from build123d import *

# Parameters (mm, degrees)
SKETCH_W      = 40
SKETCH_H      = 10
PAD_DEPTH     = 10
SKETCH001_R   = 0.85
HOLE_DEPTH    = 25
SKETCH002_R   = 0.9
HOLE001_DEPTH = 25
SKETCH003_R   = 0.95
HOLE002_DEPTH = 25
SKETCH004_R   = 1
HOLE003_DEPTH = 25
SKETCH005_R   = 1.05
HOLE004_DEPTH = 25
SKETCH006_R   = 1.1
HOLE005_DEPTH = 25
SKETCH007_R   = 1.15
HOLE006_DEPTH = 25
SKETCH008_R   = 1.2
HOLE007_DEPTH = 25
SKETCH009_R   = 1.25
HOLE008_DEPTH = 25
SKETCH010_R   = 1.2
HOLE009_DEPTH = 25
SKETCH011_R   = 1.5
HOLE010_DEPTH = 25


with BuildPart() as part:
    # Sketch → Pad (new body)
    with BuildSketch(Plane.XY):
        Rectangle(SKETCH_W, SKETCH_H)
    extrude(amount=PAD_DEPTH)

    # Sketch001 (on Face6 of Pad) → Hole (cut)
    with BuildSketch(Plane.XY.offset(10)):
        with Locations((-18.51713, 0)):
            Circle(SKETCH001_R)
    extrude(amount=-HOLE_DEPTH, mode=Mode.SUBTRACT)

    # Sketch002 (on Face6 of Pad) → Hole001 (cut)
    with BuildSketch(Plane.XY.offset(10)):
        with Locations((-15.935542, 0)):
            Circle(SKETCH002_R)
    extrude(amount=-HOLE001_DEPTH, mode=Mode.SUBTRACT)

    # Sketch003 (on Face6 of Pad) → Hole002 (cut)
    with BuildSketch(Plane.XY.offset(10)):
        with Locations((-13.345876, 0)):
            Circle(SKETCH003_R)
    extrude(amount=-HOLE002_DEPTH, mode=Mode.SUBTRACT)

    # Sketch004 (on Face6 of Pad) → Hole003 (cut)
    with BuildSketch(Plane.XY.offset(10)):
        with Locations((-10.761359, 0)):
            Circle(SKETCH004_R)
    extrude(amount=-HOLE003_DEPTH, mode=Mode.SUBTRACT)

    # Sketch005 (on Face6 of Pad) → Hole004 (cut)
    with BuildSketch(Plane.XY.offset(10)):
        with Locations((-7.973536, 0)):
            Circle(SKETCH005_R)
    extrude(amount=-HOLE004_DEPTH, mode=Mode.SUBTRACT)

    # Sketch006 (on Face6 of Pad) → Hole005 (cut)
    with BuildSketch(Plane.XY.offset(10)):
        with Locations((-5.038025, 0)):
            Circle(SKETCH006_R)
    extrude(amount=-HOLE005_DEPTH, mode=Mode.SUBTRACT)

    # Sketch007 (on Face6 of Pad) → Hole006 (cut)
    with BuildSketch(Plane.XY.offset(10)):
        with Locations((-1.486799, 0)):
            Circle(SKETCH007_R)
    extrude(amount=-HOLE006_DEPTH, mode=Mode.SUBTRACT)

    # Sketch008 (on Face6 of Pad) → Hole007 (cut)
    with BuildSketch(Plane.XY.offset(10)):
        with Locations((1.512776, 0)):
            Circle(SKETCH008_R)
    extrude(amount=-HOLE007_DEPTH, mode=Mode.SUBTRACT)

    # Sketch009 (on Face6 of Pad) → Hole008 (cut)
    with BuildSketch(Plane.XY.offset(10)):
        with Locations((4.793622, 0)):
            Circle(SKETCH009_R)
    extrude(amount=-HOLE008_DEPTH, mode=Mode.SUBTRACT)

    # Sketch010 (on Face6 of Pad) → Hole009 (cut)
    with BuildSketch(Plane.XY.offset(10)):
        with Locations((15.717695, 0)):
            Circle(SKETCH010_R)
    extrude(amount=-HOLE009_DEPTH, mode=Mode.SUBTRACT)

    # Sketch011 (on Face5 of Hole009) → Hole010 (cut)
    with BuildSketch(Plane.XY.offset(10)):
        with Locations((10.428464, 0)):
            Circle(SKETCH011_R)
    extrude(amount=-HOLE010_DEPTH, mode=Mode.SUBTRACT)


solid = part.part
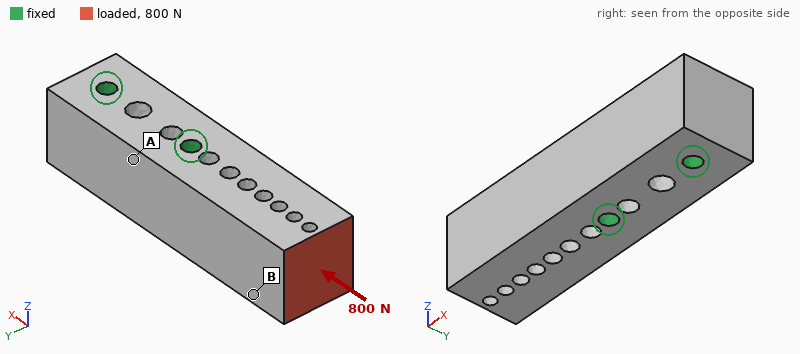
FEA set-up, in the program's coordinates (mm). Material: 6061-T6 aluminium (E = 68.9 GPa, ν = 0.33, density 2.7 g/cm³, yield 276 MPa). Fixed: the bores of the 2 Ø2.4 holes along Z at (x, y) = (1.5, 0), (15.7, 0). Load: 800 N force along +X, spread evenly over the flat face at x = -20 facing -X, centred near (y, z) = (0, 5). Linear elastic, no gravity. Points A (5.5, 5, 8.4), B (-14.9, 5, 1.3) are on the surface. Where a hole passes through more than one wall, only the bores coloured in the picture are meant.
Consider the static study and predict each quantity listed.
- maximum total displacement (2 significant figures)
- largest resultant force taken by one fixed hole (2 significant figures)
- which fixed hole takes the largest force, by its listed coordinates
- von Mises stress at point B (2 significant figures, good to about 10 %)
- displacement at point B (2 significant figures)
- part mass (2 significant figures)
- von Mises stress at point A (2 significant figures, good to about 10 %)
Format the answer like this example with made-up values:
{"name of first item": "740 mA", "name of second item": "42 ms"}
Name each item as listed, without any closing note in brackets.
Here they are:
{"maximum total displacement": "3.8 µm", "largest resultant force taken by one fixed hole": "680 N", "which fixed hole takes the largest force, by its listed coordinates": "(1.5, 0)", "von Mises stress at point B": "8.9 MPa", "displacement at point B": "2.6 µm", "part mass": "9.6 g", "von Mises stress at point A": "4.2 MPa"}
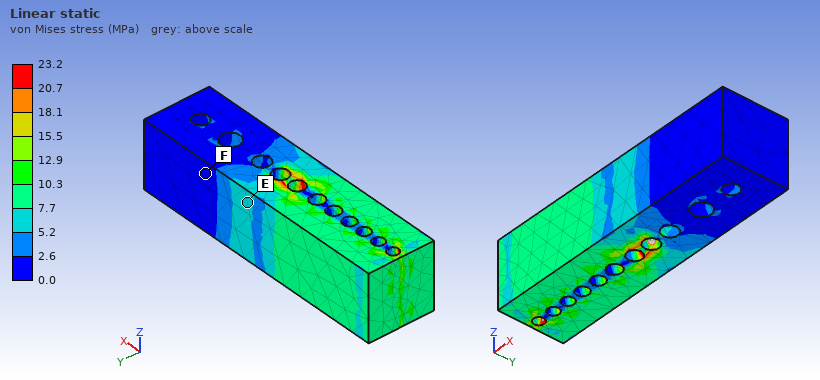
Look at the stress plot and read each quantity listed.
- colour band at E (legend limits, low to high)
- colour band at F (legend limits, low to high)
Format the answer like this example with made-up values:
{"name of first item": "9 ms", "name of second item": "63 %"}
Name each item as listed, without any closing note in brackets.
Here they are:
{"colour band at E": "5.2 to 7.7 MPa", "colour band at F": "0.0 to 2.6 MPa"}
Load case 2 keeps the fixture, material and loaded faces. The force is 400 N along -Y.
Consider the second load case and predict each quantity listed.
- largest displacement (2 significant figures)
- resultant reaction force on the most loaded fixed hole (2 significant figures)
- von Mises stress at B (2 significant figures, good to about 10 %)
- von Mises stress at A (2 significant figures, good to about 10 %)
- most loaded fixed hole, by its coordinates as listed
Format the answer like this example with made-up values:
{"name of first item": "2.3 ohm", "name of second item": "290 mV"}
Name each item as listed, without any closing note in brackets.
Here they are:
{"largest displacement": "48 µm", "resultant reaction force on the most loaded fixed hole": "770 N", "von Mises stress at B": "11 MPa", "von Mises stress at A": "26 MPa", "most loaded fixed hole, by its coordinates as listed": "(1.5, 0)"}
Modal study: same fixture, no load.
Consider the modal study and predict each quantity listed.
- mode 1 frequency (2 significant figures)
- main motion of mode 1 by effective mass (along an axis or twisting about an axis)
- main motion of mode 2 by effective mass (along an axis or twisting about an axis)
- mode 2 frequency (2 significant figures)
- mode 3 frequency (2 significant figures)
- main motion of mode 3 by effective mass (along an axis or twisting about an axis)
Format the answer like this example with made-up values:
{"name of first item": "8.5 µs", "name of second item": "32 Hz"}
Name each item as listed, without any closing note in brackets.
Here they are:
{"mode 1 frequency": "12 kHz", "main motion of mode 1 by effective mass": "along Y", "main motion of mode 2 by effective mass": "along Z", "mode 2 frequency": "13 kHz", "mode 3 frequency": "28 kHz", "main motion of mode 3 by effective mass": "twisting about X"}
